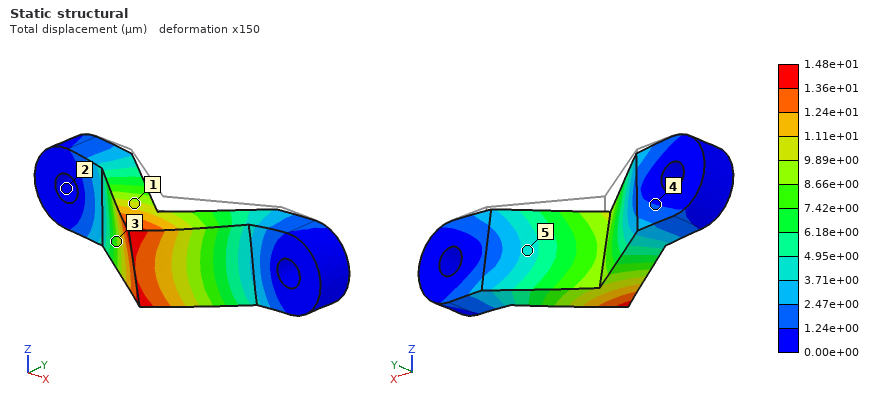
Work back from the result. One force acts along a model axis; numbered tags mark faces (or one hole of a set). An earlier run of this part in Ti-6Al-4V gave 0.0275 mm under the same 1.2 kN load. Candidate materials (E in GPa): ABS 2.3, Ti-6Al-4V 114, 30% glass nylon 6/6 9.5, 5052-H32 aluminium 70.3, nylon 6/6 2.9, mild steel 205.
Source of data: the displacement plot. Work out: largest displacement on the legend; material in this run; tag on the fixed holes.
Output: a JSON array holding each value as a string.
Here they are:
["1.48e+01 µm", "mild steel", "2"]
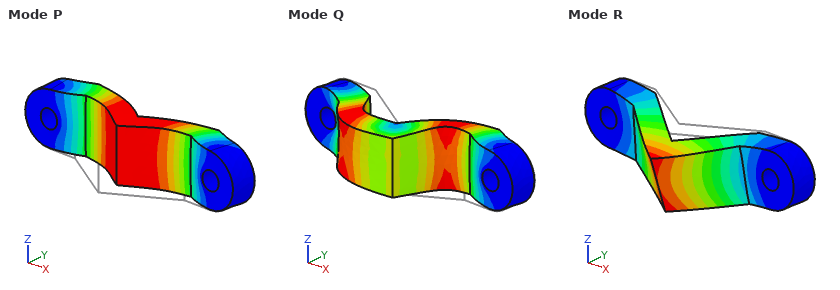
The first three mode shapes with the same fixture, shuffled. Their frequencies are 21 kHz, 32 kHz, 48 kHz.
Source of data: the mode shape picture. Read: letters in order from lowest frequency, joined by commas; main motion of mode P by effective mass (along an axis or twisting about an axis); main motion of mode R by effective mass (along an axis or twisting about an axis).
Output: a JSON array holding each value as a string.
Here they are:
["R, P, Q", "along Y", "along Z"]
